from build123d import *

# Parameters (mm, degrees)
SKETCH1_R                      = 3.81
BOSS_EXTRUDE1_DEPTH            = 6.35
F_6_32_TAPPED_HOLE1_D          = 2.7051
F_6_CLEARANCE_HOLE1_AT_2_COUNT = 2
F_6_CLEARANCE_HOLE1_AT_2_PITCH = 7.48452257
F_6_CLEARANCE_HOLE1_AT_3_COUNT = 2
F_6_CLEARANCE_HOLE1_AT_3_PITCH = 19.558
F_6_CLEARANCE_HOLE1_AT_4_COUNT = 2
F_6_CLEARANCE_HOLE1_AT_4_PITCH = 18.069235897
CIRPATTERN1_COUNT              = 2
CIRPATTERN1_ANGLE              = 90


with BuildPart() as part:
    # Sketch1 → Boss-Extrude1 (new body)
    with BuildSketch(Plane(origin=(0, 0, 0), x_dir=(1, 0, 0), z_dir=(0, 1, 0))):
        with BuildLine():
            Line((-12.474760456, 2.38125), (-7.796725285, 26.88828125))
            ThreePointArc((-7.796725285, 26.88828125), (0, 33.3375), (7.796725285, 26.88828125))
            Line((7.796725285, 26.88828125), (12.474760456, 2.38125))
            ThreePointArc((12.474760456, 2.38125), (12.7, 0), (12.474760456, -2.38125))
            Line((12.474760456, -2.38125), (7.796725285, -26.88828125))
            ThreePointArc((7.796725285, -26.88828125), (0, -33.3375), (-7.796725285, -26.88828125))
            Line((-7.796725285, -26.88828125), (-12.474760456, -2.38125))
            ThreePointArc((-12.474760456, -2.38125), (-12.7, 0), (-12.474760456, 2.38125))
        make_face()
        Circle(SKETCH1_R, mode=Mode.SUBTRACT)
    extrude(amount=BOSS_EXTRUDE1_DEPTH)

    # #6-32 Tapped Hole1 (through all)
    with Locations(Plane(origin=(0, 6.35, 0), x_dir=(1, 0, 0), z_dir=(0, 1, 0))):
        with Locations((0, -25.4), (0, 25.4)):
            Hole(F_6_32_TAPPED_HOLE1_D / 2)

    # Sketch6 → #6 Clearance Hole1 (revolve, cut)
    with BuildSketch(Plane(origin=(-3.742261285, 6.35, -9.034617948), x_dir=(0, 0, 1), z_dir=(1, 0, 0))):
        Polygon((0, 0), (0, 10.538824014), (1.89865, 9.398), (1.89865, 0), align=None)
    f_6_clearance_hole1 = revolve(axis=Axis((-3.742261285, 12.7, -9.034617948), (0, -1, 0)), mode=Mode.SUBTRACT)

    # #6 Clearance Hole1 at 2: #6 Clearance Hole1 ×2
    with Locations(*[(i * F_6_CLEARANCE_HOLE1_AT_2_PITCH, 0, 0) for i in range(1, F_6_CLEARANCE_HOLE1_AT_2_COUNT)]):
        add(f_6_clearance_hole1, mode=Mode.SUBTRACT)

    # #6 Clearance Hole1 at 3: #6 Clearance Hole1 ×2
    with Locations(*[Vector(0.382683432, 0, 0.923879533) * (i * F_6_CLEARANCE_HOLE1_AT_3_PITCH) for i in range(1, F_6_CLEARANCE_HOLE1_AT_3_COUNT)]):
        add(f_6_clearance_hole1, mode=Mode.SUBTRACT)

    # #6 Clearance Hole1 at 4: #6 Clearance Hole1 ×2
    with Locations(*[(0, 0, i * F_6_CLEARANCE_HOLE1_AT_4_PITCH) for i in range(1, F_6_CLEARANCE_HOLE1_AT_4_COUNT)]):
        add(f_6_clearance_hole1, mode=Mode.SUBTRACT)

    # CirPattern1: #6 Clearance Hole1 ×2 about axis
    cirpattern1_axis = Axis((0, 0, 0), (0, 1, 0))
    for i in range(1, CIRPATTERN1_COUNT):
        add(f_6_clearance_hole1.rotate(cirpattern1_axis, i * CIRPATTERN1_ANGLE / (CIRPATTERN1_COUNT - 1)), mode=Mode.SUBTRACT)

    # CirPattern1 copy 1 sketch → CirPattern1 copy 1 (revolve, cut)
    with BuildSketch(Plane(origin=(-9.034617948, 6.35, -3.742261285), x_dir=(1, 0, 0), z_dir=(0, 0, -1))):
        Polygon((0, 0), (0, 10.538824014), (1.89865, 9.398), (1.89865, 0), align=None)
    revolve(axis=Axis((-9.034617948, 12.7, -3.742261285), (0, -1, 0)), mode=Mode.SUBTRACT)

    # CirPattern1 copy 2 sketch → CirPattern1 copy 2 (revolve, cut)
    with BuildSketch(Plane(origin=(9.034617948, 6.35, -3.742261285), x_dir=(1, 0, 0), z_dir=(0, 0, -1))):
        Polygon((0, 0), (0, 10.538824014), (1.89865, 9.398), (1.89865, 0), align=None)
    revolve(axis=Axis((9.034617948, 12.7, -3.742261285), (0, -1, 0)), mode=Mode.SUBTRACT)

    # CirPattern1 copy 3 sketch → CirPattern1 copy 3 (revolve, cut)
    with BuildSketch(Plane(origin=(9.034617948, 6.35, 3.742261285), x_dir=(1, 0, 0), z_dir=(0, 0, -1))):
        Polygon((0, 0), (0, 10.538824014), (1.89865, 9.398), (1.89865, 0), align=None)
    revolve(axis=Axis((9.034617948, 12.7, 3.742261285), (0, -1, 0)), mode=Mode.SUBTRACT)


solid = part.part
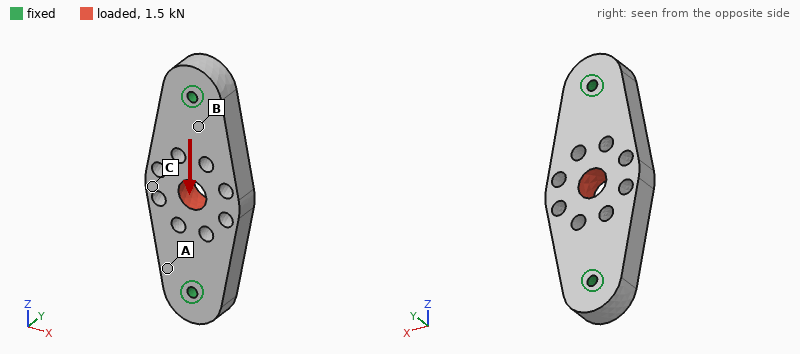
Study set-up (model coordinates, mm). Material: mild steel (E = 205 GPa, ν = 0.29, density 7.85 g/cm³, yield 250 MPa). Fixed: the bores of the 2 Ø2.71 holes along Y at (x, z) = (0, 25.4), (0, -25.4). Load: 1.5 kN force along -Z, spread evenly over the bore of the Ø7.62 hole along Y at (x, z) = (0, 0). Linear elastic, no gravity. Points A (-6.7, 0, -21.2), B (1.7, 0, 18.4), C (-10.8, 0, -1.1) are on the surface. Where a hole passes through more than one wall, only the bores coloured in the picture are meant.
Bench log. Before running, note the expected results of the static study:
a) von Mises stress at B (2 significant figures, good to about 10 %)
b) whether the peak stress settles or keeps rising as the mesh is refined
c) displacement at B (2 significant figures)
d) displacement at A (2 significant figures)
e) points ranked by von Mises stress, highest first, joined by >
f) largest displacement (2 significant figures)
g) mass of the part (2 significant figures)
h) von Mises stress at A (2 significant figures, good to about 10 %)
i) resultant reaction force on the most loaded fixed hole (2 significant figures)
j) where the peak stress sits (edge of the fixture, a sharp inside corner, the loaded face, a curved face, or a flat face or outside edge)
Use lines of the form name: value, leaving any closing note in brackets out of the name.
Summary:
von Mises stress at B: 9.1 MPa
whether the peak stress settles or keeps rising as the mesh is refined: keeps rising
displacement at B: 0.36 µm
displacement at A: 0.39 µm
points ranked by von Mises stress, highest first, joined by >: B > A > C
largest displacement: 1.2 µm
mass of the part: 56 g
von Mises stress at A: 4.8 MPa
resultant reaction force on the most loaded fixed hole: 750 N
where the peak stress sits: edge of the fixture
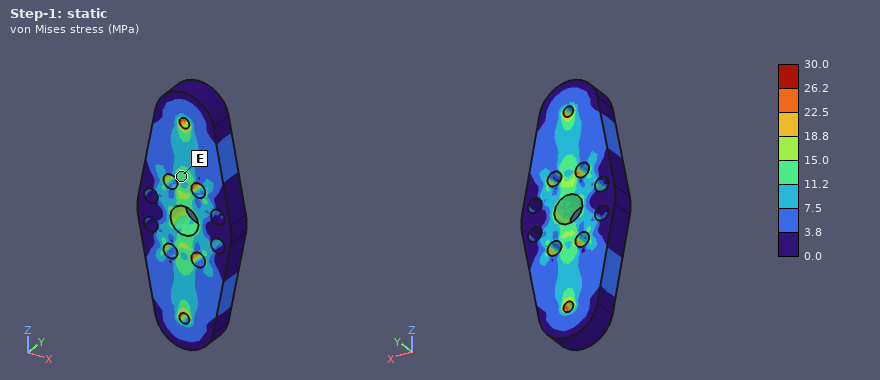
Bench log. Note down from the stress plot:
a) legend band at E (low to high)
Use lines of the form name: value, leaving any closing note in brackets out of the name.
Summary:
legend band at E: 11.2 to 15.0 MPa
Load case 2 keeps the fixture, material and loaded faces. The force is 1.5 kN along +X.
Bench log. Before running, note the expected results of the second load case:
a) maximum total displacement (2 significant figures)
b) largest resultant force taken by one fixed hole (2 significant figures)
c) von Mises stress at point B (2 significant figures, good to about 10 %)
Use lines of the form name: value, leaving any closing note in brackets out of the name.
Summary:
maximum total displacement: 6.0 µm
largest resultant force taken by one fixed hole: 750 N
von Mises stress at point B: 14 MPa
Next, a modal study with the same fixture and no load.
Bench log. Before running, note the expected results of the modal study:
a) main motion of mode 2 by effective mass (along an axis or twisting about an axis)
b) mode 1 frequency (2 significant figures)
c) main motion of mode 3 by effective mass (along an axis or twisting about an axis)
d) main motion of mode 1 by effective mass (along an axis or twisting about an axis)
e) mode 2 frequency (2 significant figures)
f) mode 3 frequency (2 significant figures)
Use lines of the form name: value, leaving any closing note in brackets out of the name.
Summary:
main motion of mode 2 by effective mass: twisting about Z
mode 1 frequency: 9600 Hz
main motion of mode 3 by effective mass: along X
main motion of mode 1 by effective mass: along Y
mode 2 frequency: 13 kHz
mode 3 frequency: 17 kHz
